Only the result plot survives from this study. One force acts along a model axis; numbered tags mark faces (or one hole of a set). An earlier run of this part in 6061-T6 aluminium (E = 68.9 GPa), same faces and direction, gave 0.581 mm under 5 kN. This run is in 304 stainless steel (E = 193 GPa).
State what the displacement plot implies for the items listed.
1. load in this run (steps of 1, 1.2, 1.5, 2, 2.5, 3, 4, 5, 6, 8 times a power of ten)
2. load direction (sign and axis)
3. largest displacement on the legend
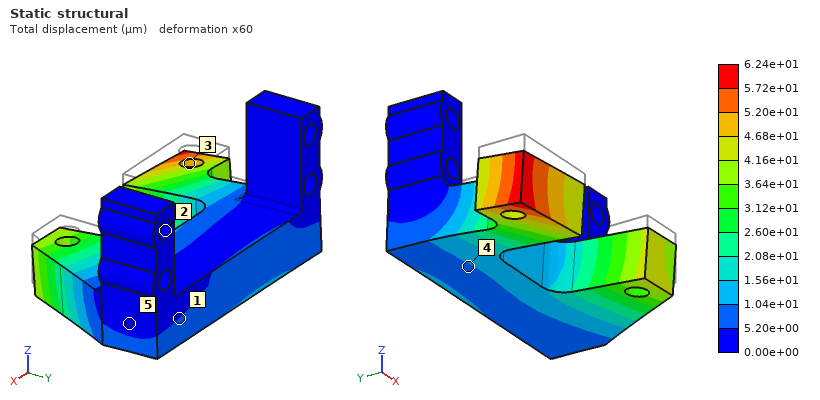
1.5 kN
-Z
6.24e+01 µm
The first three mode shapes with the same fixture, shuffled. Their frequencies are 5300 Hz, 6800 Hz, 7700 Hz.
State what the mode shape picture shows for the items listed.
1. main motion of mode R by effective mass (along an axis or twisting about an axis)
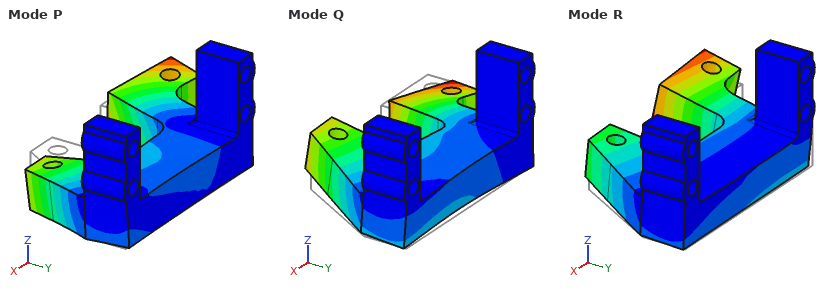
along Z
